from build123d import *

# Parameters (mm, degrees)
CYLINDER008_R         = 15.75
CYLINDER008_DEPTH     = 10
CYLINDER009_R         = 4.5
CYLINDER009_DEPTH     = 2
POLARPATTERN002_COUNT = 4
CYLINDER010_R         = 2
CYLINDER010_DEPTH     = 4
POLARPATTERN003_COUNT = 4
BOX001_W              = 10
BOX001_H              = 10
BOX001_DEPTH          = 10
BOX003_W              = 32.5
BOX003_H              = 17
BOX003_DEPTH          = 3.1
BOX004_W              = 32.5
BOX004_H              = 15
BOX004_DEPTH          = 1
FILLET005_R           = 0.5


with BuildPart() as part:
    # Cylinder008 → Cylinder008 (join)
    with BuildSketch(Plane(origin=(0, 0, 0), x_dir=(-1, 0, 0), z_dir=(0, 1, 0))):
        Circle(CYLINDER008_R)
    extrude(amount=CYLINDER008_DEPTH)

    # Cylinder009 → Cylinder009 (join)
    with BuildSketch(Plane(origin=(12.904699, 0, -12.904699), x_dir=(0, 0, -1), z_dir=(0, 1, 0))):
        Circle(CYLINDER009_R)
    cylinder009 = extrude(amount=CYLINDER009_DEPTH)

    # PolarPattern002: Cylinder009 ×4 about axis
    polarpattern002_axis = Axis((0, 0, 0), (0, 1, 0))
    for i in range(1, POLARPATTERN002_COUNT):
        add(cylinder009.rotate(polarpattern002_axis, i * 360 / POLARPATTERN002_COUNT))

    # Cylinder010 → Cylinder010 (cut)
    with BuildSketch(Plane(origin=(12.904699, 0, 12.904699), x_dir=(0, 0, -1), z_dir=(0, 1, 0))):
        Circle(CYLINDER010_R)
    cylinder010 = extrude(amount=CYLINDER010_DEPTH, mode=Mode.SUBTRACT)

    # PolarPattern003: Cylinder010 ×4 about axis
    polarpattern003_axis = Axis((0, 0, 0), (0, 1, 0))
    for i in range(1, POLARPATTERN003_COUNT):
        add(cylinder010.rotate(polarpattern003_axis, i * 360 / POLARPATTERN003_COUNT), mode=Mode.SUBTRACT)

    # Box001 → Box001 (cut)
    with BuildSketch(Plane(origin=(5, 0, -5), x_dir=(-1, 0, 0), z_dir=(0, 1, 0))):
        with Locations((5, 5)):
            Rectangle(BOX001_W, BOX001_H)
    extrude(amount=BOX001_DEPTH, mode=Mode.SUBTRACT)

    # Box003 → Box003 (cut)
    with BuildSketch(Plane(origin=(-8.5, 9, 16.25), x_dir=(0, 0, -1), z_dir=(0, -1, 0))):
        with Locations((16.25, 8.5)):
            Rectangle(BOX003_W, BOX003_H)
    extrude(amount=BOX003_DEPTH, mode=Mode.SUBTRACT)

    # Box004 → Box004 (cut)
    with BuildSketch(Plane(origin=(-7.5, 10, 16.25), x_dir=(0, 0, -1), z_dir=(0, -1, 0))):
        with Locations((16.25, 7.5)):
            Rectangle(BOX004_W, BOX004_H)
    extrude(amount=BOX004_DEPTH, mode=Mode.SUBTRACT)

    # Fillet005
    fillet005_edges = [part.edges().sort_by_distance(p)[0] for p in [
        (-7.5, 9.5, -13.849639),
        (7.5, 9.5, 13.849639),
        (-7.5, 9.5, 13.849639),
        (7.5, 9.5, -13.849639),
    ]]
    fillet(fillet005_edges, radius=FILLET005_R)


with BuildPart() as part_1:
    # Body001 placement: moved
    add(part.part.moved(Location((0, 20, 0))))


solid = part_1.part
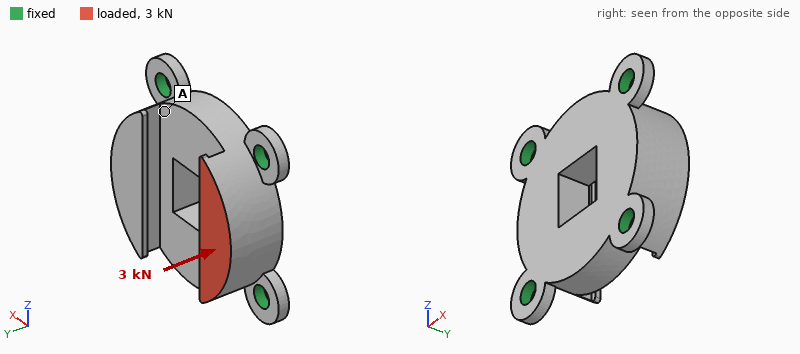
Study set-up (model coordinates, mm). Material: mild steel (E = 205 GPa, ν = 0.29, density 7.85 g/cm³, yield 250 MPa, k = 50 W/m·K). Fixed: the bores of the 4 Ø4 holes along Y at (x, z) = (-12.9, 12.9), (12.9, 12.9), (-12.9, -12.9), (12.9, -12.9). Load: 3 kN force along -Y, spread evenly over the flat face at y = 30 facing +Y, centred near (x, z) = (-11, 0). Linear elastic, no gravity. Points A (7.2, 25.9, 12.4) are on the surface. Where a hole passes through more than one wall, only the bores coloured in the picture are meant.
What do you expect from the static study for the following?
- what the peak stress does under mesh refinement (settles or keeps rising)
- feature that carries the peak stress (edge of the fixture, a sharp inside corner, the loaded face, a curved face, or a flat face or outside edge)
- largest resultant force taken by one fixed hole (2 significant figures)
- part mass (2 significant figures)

keeps rising
edge of the fixture
1.6 kN
43 g
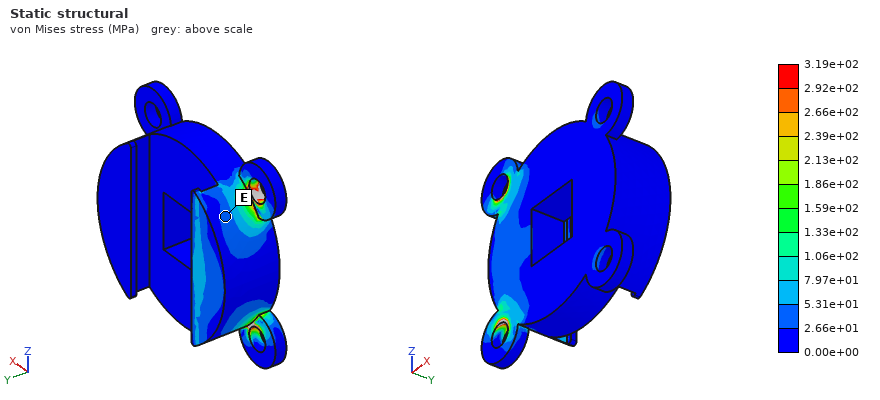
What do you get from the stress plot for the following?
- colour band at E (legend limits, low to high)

2.66e+01 to 5.31e+01 MPa
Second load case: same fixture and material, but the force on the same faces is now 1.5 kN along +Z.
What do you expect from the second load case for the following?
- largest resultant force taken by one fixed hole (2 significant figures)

840 N
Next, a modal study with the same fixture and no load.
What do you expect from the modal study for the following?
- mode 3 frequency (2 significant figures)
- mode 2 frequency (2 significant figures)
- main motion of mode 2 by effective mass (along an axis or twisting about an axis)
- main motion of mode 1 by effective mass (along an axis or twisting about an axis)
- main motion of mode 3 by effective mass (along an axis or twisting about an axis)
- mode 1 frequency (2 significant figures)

27 kHz
26 kHz
along X
along Y
along Y
21 kHz
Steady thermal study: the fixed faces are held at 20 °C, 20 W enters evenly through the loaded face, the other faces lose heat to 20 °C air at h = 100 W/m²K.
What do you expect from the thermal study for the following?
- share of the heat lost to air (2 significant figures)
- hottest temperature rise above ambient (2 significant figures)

22 %
49 K
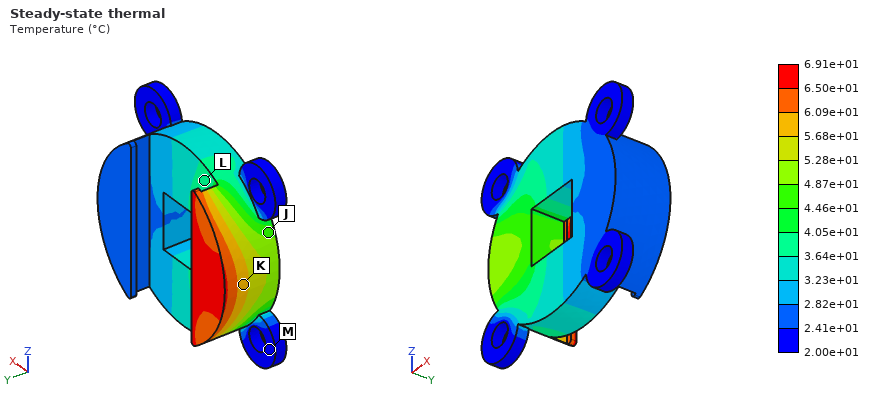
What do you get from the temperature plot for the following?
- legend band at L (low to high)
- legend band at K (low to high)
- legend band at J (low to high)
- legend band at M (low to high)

3.64e+01 to 4.05e+01 °C
5.68e+01 to 6.09e+01 °C
4.46e+01 to 4.87e+01 °C
2.00e+01 to 2.41e+01 °C
